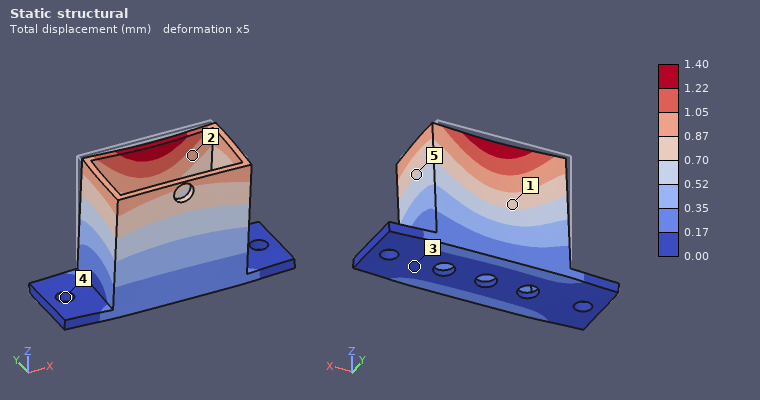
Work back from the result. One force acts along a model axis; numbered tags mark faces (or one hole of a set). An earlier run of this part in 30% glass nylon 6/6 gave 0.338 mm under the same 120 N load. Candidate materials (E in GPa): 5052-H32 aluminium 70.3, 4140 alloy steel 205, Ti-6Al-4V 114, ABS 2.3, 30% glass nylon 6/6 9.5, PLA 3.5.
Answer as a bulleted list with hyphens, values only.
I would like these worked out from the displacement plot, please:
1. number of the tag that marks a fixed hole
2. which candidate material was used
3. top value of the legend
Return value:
- 4
- ABS
- 1.40 mm
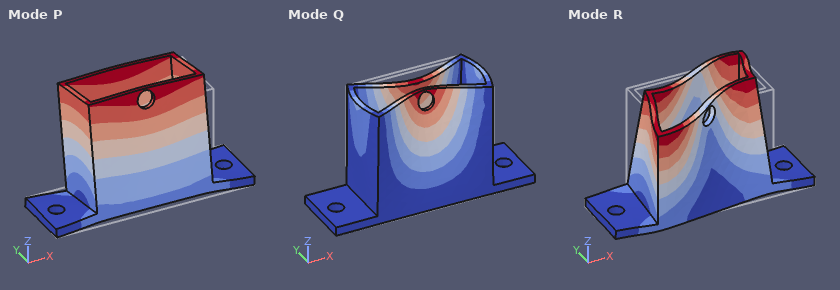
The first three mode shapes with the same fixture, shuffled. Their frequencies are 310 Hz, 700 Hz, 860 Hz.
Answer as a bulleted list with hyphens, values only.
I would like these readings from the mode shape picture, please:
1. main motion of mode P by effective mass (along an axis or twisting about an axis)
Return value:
- along Y
